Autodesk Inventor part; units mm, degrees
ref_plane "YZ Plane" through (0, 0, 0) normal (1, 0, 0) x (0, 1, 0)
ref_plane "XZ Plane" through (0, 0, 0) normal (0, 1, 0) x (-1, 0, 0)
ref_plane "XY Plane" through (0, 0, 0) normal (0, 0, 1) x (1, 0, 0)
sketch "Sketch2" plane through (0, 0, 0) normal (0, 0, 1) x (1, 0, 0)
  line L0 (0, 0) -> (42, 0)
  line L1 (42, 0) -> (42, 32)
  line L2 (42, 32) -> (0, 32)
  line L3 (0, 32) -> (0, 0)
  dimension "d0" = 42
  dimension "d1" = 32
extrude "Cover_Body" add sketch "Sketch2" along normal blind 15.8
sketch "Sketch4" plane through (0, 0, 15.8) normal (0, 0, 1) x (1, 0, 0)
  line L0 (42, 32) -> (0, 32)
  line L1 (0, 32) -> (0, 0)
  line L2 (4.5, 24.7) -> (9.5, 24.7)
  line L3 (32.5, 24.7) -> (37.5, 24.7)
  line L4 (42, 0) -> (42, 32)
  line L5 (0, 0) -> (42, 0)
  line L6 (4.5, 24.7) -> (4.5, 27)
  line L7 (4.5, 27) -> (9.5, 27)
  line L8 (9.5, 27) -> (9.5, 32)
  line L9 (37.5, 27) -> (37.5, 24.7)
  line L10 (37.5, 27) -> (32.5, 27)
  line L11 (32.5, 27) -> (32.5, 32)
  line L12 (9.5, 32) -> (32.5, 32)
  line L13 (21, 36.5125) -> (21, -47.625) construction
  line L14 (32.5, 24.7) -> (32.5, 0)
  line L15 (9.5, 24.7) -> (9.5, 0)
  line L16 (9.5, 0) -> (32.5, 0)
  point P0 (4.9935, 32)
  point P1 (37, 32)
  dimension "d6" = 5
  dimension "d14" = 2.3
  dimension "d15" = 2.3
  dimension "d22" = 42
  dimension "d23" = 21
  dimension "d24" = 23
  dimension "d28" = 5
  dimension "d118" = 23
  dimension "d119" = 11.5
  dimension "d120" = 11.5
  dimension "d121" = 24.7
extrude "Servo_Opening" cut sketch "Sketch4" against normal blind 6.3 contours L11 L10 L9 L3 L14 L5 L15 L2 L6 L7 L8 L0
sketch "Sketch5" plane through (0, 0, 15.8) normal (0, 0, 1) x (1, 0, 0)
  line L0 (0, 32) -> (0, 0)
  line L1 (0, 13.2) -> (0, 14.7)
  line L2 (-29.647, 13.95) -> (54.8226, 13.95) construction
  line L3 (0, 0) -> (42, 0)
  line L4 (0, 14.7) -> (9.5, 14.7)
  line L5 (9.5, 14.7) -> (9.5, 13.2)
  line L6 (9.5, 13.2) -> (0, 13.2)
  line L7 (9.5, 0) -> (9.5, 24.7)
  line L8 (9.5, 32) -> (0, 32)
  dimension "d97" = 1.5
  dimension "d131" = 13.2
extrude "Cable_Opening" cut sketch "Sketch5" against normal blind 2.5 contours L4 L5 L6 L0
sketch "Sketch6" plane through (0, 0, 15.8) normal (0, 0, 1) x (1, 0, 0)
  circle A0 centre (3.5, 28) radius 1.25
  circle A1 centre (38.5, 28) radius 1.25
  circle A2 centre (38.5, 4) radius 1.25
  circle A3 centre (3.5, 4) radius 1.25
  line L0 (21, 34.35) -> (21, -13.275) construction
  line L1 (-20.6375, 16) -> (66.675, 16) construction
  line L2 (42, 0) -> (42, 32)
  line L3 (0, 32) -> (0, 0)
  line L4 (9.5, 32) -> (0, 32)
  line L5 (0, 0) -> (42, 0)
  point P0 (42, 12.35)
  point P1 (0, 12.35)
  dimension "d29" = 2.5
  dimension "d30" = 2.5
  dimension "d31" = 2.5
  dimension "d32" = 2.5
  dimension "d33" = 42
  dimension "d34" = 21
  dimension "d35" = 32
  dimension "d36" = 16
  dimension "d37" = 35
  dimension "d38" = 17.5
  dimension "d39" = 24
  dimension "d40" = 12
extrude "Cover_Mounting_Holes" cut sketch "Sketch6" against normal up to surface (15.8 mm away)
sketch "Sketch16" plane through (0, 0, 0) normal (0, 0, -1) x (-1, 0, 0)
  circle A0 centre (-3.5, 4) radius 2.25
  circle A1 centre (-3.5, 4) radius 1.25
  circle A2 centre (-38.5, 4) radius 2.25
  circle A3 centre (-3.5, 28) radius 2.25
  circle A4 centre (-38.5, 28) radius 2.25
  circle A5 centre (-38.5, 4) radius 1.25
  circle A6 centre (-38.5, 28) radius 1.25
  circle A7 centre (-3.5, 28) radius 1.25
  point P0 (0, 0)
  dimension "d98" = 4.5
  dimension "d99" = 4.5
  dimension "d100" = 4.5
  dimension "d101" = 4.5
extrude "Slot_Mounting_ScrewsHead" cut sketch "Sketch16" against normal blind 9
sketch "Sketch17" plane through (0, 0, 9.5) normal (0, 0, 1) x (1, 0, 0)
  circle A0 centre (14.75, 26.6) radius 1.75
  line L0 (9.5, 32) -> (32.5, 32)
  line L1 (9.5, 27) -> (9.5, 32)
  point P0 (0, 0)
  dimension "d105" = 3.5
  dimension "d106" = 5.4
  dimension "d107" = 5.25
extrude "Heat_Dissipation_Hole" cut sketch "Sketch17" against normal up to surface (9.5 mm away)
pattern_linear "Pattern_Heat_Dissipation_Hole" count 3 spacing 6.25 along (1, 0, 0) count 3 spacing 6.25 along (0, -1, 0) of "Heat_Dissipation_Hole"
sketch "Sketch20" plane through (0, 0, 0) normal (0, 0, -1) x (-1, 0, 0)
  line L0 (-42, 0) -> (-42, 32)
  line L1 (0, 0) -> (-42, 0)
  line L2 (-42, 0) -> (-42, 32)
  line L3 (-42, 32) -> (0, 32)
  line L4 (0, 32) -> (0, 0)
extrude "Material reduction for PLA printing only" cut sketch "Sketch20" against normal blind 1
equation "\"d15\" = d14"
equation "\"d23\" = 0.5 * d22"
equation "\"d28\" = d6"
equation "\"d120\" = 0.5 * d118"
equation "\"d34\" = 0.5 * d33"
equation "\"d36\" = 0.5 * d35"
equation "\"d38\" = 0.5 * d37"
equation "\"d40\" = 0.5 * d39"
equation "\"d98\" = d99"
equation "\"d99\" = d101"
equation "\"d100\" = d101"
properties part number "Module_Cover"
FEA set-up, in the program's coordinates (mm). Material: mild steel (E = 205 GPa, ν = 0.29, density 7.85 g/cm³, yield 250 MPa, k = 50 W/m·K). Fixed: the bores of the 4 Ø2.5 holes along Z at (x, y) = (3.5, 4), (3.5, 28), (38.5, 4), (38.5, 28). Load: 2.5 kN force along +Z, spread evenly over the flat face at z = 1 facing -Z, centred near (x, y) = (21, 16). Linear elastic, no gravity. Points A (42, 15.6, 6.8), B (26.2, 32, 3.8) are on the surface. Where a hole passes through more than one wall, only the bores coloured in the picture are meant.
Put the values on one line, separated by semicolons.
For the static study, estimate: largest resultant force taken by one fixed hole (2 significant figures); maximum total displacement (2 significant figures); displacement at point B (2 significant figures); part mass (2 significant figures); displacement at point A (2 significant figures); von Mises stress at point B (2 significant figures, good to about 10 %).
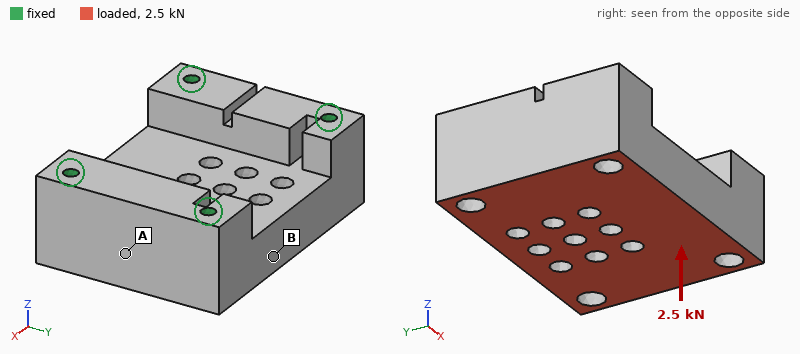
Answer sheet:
770 N; 1.8 µm; 1.4 µm; 110 g; 0.39 µm; 6.8 MPa
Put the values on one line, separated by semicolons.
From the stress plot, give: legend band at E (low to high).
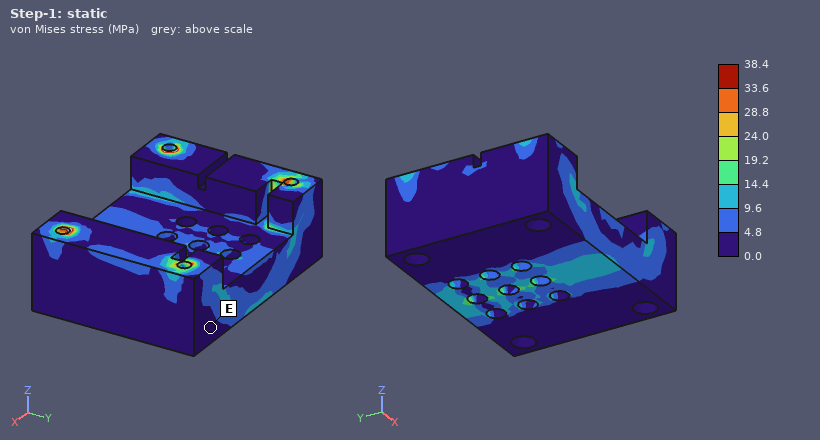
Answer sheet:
0.0 to 4.8 MPa
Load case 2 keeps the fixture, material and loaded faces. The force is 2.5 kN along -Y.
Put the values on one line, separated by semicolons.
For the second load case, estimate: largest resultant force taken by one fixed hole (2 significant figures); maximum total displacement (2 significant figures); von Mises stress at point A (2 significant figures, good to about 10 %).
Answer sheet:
880 N; 2.0 µm; 8.3 MPa
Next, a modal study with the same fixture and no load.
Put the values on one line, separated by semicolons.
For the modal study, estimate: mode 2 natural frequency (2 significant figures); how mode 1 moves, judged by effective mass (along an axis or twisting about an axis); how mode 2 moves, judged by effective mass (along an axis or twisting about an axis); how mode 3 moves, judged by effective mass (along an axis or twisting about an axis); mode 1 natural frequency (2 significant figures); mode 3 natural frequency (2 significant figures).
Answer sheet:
26 kHz; along Z; along X; along Y; 23 kHz; 28 kHz
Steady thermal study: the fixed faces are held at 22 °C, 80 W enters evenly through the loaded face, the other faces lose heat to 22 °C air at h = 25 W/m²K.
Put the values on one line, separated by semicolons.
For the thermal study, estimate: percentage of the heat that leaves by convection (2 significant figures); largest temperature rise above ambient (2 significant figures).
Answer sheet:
4.4 %; 50 K
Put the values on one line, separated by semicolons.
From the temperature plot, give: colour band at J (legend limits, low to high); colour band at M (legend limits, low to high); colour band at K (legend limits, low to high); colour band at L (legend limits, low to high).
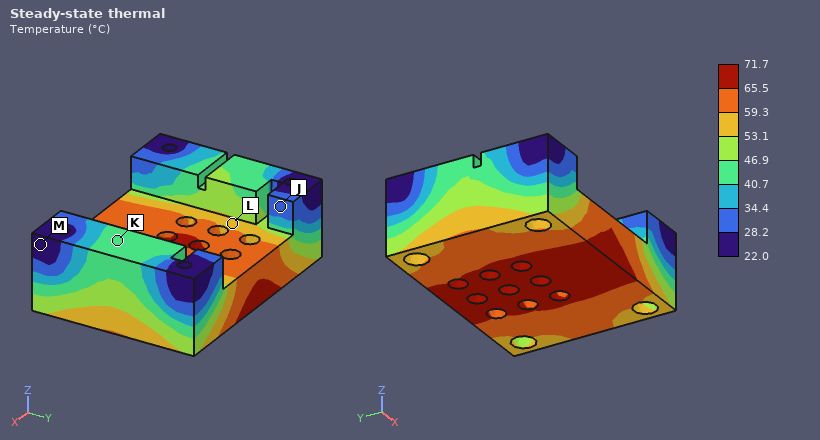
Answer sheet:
28.2 to 34.4 °C; 22.0 to 28.2 °C; 40.7 to 46.9 °C; 53.1 to 59.3 °C
